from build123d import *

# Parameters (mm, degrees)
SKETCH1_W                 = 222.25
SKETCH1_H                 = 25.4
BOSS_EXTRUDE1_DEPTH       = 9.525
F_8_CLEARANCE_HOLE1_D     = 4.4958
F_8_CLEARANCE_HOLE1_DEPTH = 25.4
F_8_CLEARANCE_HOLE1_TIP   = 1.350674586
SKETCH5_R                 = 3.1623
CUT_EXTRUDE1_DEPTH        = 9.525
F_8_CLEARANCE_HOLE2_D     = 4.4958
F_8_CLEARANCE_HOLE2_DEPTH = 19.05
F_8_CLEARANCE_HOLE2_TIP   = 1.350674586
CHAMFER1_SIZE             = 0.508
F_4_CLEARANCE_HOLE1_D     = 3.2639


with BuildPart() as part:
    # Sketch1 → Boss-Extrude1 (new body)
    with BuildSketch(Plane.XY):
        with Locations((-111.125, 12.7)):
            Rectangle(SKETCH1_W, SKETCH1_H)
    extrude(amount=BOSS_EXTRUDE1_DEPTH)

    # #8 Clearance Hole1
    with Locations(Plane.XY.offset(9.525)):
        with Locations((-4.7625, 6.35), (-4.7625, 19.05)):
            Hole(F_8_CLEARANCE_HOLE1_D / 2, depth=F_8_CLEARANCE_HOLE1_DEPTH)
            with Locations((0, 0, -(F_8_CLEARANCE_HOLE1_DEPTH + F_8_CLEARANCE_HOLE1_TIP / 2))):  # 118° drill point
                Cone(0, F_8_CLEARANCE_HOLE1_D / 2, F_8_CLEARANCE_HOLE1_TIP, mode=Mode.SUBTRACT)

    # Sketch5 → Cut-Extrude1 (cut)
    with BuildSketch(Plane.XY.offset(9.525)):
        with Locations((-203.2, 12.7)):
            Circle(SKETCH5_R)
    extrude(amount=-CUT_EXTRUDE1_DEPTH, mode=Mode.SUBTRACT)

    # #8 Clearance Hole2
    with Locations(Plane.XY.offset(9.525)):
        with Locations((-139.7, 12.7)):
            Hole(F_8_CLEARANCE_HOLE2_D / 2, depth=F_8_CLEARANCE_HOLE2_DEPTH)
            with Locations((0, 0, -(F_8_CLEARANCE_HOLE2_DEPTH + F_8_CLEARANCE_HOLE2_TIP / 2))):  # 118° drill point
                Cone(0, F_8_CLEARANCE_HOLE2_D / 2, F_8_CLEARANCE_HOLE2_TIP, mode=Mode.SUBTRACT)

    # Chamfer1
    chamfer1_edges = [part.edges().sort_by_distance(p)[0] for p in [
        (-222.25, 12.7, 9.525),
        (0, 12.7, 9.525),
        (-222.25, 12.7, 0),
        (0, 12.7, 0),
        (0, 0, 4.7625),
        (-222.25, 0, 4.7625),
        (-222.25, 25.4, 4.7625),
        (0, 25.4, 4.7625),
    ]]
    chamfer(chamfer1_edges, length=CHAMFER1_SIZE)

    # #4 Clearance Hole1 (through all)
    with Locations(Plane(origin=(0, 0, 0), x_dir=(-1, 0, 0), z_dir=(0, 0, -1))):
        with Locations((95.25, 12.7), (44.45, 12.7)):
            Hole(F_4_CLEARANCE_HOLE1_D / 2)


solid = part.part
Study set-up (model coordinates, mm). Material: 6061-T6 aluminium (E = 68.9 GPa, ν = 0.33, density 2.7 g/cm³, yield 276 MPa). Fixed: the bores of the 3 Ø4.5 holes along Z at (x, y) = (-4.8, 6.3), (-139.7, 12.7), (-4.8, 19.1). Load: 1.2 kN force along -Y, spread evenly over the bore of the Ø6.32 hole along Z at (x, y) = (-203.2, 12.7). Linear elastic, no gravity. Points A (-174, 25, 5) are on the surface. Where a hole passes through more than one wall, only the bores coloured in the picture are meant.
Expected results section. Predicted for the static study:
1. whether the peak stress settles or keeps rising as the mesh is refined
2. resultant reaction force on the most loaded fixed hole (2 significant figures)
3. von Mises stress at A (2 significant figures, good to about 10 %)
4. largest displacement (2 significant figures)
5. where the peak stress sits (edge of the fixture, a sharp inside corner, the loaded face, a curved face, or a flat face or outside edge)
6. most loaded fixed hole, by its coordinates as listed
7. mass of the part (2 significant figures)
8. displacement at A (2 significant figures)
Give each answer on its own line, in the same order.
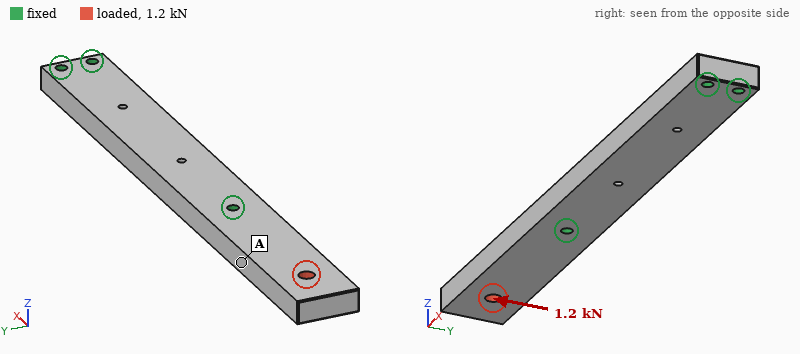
keeps rising
1.7 kN
34 MPa
0.34 mm
edge of the fixture
(-139.7, 12.7)
140 g
0.12 mm
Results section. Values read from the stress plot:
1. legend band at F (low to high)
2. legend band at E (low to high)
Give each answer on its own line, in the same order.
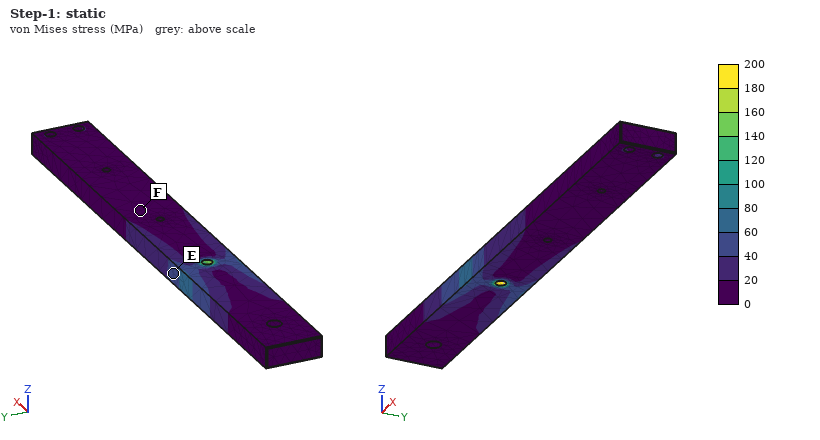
0 to 20 MPa
40 to 60 MPa
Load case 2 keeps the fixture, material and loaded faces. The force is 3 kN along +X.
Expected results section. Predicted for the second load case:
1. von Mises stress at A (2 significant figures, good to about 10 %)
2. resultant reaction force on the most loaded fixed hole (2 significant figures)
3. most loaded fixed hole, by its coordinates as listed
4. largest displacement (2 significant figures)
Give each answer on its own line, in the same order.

13 MPa
2.9 kN
(-139.7, 12.7)
14 µm
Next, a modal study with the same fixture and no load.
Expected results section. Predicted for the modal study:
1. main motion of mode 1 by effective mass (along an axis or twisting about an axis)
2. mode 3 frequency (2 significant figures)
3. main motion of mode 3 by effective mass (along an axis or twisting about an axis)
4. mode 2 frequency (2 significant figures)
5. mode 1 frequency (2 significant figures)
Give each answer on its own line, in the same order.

along Z
2600 Hz
along Z
2000 Hz
1100 Hz
